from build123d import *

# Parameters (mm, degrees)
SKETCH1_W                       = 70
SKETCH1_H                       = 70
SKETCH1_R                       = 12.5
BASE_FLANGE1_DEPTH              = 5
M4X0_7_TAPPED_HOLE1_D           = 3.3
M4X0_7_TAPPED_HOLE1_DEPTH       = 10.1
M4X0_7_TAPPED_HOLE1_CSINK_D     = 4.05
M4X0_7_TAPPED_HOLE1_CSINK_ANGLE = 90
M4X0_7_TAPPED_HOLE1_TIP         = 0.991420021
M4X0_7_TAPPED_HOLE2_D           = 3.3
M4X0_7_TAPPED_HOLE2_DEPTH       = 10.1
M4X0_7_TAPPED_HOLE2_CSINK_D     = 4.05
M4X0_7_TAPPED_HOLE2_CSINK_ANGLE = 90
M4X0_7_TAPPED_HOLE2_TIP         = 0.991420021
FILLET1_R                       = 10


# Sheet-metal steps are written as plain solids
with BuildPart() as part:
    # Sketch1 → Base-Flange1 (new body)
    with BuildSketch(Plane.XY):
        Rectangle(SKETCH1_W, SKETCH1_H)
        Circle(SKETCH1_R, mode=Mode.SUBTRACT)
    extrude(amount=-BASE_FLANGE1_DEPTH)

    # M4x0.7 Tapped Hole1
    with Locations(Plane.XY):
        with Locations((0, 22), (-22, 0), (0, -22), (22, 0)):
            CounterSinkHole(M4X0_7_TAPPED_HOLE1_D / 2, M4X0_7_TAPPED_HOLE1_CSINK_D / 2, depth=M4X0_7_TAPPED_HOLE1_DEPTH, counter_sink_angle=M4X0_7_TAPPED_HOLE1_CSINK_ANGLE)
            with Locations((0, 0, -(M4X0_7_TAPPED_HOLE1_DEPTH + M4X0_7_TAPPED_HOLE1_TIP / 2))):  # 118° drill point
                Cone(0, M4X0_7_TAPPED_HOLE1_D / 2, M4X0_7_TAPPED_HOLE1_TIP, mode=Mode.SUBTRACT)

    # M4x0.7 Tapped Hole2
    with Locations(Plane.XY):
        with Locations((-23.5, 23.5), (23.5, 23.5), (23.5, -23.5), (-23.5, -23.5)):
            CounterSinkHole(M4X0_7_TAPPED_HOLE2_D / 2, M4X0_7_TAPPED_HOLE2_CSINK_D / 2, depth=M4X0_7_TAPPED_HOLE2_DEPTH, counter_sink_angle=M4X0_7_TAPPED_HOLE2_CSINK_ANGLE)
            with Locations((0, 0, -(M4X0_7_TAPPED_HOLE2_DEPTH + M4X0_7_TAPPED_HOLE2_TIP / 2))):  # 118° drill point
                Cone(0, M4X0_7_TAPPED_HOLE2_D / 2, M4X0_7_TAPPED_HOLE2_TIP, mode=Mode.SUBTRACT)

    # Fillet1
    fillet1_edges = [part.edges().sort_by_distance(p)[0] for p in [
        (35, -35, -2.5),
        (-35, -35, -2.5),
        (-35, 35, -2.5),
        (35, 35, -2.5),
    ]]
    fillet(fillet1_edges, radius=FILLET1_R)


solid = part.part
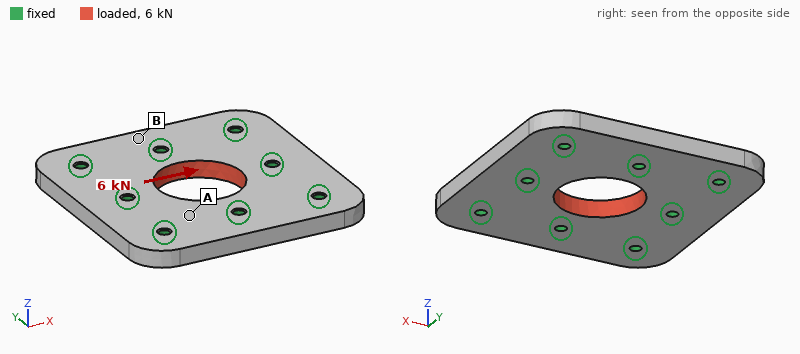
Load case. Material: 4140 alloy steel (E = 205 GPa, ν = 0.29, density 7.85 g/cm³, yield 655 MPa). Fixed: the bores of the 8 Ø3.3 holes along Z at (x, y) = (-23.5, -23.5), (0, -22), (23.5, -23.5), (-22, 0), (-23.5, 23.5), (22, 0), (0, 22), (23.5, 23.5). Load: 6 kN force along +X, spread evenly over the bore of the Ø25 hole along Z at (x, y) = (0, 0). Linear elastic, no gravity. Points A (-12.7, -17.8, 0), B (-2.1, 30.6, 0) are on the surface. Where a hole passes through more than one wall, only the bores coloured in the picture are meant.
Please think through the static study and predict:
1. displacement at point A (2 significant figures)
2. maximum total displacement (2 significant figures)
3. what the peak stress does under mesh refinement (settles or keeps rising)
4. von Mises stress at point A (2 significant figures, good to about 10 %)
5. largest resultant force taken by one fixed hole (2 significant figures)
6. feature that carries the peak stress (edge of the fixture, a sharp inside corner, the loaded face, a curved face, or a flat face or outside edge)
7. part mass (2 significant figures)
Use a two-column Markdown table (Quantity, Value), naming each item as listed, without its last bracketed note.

| Quantity | Value |
|---|---|
| displacement at point A | 0.51 µm |
| maximum total displacement | 1.4 µm |
| what the peak stress does under mesh refinement | keeps rising |
| von Mises stress at point A | 9.7 MPa |
| largest resultant force taken by one fixed hole | 1.3 kN |
| feature that carries the peak stress | edge of the fixture |
| part mass | 170 g |
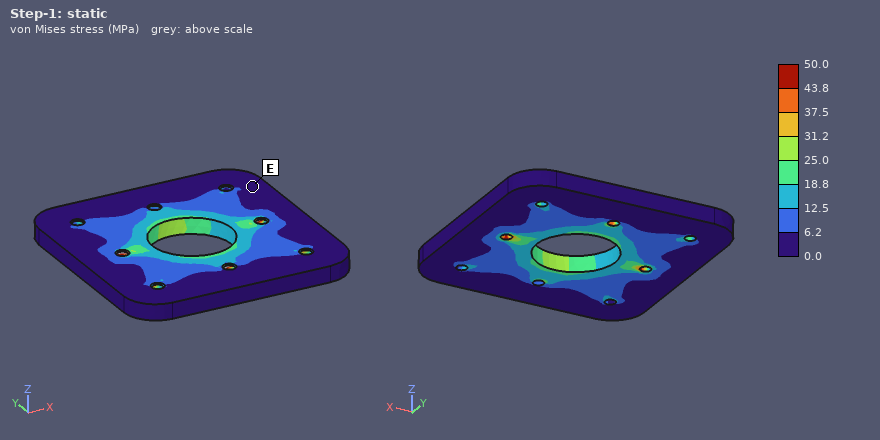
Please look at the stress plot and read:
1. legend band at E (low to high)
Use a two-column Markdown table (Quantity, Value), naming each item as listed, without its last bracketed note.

| Quantity | Value |
|---|---|
| legend band at E | 0.0 to 6.2 MPa |
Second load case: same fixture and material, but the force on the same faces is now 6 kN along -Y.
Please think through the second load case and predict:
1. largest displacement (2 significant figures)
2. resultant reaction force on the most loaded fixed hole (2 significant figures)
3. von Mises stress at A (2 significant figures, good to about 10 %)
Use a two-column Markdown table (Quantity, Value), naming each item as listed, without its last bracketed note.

| Quantity | Value |
|---|---|
| largest displacement | 1.4 µm |
| resultant reaction force on the most loaded fixed hole | 1.3 kN |
| von Mises stress at A | 9.1 MPa |
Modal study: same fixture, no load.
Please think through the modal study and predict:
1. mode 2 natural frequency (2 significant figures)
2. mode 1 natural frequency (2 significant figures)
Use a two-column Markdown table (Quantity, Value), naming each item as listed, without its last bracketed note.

| Quantity | Value |
|---|---|
| mode 2 natural frequency | 20 kHz |
| mode 1 natural frequency | 20 kHz |
